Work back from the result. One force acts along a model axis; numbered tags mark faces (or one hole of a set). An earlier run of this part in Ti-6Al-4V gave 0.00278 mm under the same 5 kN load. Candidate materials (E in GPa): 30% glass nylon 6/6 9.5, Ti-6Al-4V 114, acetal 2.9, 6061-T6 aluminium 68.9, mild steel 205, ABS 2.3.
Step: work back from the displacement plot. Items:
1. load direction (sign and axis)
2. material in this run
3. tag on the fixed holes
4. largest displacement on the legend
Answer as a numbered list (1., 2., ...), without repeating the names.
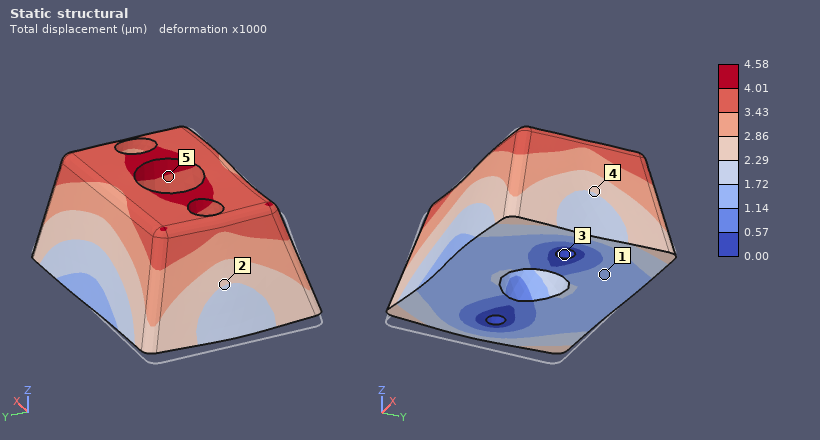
1. +X
2. 6061-T6 aluminium
3. 3
4. 4.58 µm
